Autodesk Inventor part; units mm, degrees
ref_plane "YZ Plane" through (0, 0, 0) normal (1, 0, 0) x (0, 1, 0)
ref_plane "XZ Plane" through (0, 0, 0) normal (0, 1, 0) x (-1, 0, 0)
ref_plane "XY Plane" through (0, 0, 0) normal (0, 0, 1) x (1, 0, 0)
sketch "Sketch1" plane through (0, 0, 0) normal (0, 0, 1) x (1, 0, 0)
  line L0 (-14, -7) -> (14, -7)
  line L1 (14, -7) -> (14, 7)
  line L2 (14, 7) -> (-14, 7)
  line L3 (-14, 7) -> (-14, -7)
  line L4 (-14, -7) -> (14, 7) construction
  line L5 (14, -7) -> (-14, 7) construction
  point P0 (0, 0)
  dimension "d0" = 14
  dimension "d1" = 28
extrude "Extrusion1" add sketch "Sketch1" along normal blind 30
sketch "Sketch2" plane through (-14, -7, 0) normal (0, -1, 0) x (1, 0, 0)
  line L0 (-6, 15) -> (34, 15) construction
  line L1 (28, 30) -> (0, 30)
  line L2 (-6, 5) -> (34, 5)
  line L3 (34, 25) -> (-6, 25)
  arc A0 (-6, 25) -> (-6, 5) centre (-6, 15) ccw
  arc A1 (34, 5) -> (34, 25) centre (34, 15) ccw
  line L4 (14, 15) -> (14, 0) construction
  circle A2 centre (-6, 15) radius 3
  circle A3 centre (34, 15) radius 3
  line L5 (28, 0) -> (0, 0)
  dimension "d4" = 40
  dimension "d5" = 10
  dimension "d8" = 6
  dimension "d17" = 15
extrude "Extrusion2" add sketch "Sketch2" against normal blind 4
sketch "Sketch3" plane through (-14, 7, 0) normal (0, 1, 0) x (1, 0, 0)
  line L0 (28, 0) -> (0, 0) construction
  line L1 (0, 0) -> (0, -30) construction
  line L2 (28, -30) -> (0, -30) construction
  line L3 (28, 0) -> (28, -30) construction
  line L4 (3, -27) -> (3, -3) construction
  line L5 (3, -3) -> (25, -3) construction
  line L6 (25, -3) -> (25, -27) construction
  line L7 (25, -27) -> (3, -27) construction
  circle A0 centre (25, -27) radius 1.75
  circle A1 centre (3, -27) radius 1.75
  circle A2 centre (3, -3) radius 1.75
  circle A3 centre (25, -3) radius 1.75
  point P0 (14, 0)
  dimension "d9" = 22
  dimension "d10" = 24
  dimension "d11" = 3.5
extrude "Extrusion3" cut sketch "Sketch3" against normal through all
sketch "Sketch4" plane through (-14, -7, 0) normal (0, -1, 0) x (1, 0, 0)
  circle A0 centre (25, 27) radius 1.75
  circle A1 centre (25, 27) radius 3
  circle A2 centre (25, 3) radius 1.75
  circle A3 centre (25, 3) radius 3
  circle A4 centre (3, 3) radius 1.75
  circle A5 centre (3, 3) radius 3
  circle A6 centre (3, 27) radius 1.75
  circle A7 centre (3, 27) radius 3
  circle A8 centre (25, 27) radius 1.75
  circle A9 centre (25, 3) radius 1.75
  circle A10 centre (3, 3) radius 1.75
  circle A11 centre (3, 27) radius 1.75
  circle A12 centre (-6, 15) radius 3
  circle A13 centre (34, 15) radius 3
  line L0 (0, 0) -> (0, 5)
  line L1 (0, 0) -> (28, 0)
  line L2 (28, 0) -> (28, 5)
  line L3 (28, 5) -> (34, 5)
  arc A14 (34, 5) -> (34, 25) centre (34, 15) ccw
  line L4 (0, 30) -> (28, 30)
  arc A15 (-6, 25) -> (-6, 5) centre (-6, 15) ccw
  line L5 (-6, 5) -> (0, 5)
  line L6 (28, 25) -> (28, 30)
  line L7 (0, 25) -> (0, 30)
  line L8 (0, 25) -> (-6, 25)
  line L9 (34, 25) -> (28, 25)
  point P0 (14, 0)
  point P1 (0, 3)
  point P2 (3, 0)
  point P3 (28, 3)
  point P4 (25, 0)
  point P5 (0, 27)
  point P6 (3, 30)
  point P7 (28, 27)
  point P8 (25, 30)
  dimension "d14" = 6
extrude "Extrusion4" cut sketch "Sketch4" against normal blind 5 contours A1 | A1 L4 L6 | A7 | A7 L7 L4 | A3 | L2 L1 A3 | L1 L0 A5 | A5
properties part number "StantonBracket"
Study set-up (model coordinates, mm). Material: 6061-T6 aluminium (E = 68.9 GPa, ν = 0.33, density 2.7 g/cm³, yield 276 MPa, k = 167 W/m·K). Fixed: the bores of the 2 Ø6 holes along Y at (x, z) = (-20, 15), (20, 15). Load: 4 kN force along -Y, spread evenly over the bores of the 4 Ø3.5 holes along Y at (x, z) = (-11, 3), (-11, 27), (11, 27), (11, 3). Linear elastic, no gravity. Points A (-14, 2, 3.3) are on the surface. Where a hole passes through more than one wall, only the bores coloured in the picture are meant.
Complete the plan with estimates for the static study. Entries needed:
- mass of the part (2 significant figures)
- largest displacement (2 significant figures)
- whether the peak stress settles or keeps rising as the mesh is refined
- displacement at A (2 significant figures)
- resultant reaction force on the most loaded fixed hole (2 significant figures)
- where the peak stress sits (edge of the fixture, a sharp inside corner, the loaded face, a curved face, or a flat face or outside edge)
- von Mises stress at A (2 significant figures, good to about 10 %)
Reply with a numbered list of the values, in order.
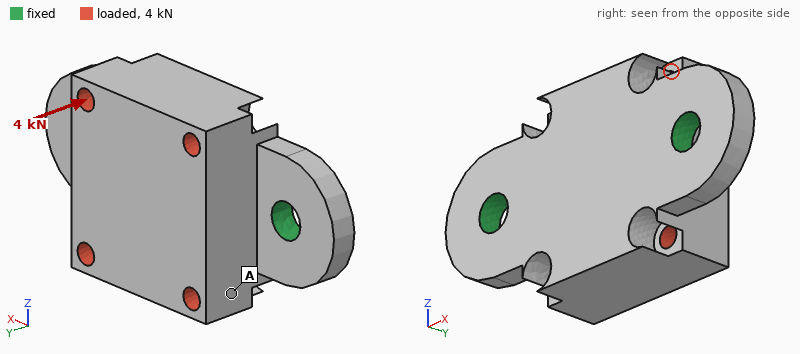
1. 35 g
2. 25 µm
3. keeps rising
4. 22 µm
5. 2.3 kN
6. edge of the fixture
7. 38 MPa
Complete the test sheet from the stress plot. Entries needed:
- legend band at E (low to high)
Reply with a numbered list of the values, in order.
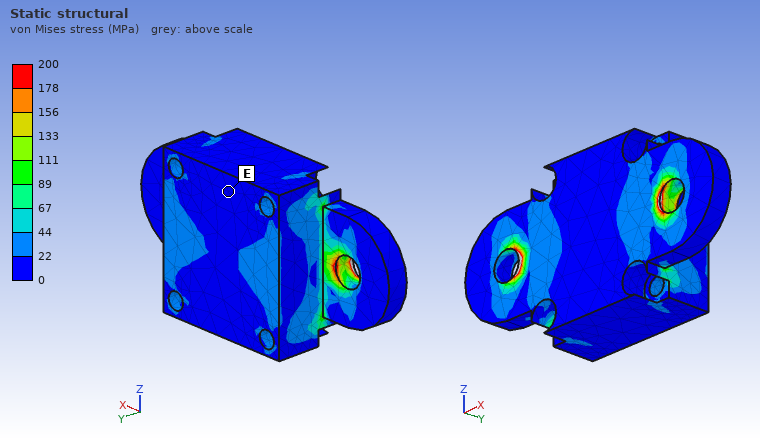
1. 0 to 22 MPa
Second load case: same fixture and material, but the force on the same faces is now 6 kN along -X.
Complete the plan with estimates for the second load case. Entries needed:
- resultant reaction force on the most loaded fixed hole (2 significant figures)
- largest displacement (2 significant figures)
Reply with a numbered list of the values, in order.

1. 3.3 kN
2. 22 µm
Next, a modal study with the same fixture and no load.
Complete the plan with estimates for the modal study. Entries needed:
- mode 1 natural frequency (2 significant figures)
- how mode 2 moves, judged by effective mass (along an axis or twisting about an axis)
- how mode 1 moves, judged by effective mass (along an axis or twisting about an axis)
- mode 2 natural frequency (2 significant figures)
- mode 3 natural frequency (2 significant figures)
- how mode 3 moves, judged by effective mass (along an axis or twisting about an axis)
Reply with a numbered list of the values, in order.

1. 6200 Hz
2. along Y
3. along Z
4. 13 kHz
5. 20 kHz
6. along Z
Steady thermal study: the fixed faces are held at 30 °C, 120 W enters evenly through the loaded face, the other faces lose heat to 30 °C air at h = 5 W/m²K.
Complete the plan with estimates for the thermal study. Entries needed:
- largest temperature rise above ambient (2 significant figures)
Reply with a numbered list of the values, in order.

1. 59 K
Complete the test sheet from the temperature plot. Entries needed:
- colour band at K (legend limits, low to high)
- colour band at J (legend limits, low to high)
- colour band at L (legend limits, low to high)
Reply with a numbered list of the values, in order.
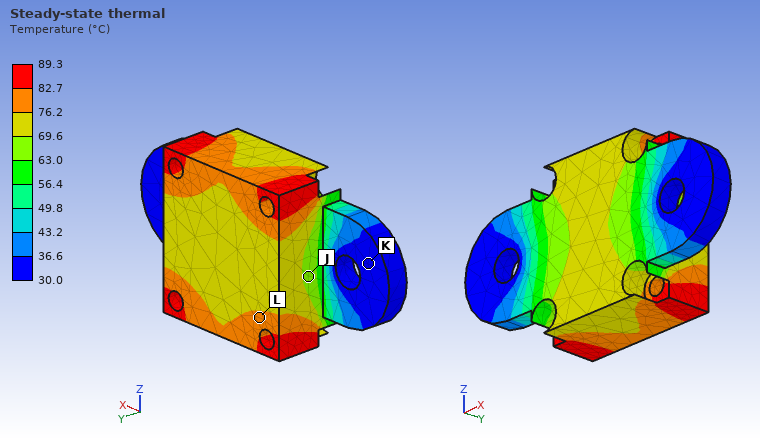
1. 30.0 to 36.6 °C
2. 63.0 to 69.6 °C
3. 76.2 to 82.7 °C
